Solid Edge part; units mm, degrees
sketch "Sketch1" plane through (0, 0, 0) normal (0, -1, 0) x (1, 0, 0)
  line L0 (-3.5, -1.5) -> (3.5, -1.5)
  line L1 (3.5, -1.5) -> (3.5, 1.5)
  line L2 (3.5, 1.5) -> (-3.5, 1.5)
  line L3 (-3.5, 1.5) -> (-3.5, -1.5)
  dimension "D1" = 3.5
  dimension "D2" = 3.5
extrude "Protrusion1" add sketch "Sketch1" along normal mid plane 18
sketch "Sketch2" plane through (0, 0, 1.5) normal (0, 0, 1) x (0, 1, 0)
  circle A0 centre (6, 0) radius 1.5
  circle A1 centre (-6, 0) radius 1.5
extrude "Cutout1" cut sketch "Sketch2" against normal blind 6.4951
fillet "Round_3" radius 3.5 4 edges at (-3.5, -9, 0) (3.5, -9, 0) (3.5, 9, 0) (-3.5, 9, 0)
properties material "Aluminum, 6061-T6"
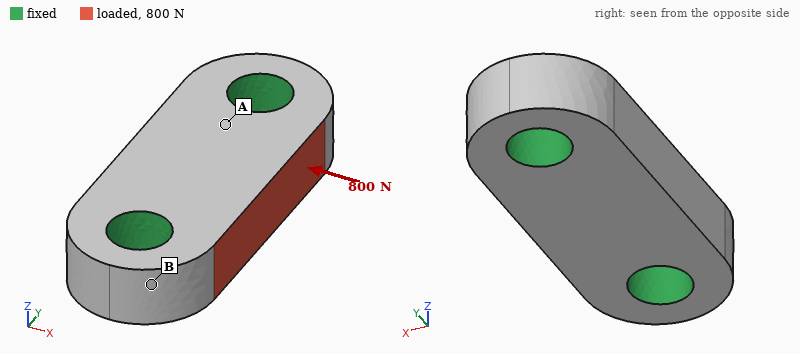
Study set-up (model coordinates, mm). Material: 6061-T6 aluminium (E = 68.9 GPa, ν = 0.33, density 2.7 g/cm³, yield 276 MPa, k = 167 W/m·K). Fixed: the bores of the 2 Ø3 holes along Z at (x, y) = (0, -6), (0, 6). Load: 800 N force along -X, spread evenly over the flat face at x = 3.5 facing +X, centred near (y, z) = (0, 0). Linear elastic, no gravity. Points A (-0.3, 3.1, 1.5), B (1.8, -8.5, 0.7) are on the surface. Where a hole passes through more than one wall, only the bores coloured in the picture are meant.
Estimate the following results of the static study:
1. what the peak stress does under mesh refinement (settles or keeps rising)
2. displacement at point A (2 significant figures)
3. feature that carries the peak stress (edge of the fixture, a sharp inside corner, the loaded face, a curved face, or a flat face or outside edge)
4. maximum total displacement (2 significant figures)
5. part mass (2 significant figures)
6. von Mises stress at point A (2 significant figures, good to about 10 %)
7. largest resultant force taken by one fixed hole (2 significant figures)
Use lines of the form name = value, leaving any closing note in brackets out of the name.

what the peak stress does under mesh refinement = keeps rising
displacement at point A = 1.5 µm
feature that carries the peak stress = edge of the fixture
maximum total displacement = 3.5 µm
part mass = 0.82 g
von Mises stress at point A = 27 MPa
largest resultant force taken by one fixed hole = 410 N
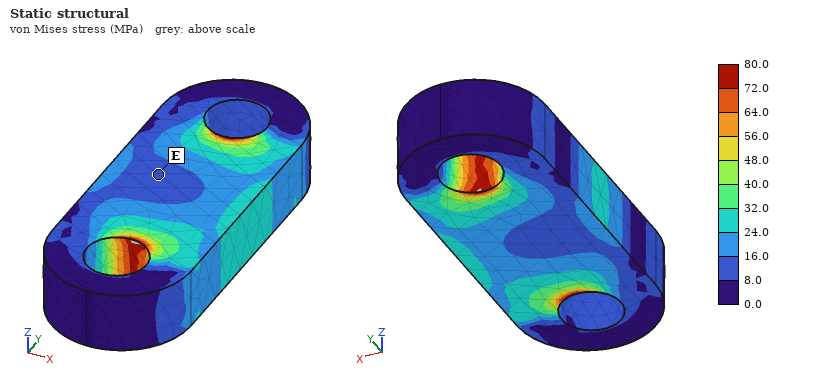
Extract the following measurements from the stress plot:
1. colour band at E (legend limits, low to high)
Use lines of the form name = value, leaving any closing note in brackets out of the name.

colour band at E = 8.0 to 16.0 MPa
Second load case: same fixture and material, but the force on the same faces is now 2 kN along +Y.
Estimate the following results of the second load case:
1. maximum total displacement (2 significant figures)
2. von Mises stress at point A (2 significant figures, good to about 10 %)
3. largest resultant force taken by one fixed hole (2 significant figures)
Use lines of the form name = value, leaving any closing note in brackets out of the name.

maximum total displacement = 6.8 µm
von Mises stress at point A = 33 MPa
largest resultant force taken by one fixed hole = 1.1 kN
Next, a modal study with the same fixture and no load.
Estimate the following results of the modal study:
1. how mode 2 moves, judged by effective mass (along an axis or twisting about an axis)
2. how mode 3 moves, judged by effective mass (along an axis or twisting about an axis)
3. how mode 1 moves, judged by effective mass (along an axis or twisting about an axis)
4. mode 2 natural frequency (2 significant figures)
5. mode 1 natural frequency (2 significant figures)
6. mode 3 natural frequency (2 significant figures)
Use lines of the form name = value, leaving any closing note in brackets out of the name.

how mode 2 moves, judged by effective mass = twisting about Y
how mode 3 moves, judged by effective mass = along X
how mode 1 moves, judged by effective mass = along Z
mode 2 natural frequency = 110 kHz
mode 1 natural frequency = 98 kHz
mode 3 natural frequency = 120 kHz
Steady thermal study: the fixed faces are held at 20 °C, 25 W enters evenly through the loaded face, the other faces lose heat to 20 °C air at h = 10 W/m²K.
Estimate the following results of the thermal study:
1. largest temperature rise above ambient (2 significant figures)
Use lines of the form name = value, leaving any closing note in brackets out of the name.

largest temperature rise above ambient = 19 K
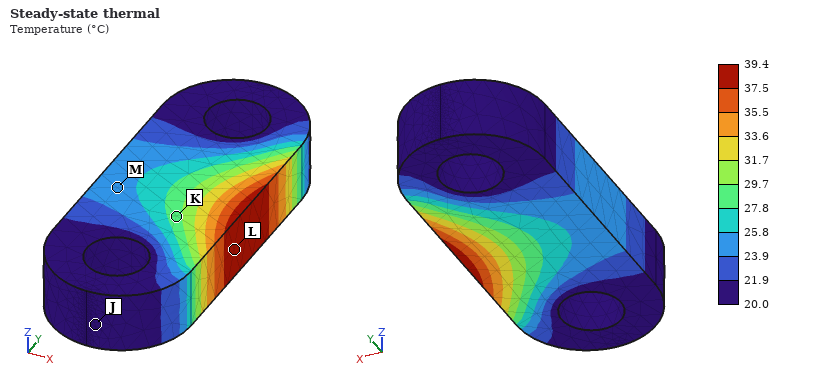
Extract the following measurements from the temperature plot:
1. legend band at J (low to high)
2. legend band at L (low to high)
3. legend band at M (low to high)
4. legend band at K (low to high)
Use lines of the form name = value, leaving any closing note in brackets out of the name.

legend band at J = 20.0 to 21.9 °C
legend band at L = 37.5 to 39.4 °C
legend band at M = 23.9 to 25.8 °C
legend band at K = 27.8 to 29.7 °C
